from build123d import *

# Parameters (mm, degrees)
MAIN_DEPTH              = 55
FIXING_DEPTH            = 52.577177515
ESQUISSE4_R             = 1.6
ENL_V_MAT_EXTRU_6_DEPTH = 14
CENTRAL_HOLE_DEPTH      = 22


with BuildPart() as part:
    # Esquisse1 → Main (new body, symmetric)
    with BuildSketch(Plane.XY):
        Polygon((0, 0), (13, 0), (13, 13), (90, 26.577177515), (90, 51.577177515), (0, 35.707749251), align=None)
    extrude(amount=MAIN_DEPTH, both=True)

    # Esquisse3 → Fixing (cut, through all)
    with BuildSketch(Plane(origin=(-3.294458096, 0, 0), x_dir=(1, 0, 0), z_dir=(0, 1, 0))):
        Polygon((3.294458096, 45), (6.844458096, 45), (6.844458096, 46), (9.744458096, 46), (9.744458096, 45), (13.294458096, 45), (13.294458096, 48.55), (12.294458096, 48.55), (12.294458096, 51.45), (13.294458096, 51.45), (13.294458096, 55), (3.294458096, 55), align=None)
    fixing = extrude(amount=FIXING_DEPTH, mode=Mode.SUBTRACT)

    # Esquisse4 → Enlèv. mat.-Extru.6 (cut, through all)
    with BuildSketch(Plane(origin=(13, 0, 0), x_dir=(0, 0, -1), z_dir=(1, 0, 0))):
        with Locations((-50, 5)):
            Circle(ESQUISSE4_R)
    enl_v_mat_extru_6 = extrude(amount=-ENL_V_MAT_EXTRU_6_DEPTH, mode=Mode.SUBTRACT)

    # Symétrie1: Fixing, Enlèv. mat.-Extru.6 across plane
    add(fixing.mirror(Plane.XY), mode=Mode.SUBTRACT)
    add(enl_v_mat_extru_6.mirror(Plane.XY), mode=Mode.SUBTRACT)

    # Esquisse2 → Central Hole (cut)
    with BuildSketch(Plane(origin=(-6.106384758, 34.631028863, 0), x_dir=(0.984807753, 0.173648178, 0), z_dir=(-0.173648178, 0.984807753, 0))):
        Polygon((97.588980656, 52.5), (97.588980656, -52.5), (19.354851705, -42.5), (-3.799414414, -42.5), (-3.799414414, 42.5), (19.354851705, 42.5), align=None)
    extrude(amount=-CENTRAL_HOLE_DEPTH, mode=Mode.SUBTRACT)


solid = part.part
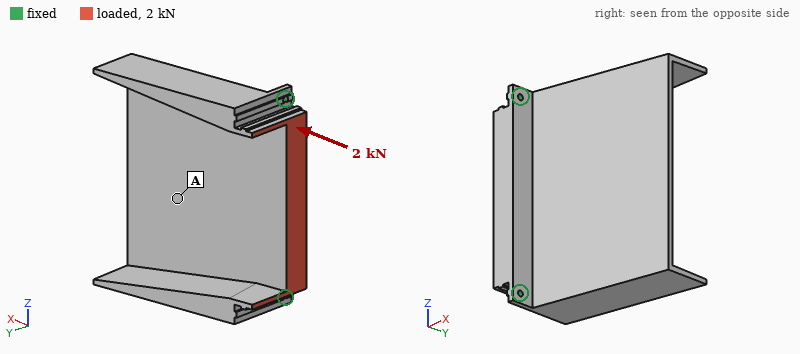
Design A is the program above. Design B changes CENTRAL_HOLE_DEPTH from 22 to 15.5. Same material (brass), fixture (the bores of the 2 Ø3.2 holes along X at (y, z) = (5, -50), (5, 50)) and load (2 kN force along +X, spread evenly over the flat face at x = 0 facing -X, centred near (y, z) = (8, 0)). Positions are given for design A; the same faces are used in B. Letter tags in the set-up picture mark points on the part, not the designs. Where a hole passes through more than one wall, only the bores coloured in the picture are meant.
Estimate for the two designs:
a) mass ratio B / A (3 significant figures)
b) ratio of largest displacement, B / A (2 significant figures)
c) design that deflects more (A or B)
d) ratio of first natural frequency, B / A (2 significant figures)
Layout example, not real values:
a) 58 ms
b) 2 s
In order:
a) 1.79
b) 2.2
c) B
d) 0.73
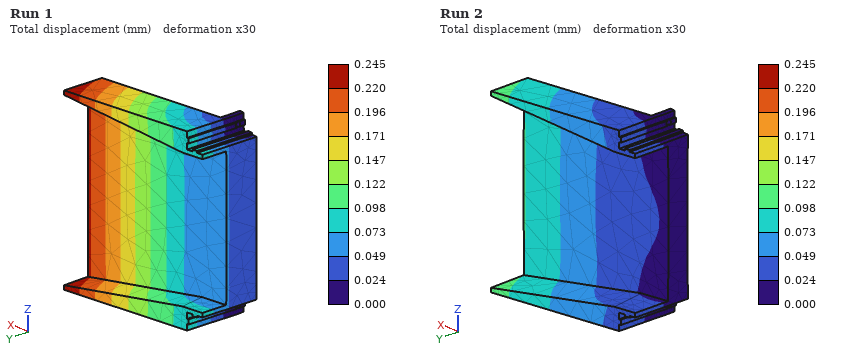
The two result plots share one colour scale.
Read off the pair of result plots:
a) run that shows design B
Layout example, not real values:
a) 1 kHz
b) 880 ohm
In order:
a) Run 1
